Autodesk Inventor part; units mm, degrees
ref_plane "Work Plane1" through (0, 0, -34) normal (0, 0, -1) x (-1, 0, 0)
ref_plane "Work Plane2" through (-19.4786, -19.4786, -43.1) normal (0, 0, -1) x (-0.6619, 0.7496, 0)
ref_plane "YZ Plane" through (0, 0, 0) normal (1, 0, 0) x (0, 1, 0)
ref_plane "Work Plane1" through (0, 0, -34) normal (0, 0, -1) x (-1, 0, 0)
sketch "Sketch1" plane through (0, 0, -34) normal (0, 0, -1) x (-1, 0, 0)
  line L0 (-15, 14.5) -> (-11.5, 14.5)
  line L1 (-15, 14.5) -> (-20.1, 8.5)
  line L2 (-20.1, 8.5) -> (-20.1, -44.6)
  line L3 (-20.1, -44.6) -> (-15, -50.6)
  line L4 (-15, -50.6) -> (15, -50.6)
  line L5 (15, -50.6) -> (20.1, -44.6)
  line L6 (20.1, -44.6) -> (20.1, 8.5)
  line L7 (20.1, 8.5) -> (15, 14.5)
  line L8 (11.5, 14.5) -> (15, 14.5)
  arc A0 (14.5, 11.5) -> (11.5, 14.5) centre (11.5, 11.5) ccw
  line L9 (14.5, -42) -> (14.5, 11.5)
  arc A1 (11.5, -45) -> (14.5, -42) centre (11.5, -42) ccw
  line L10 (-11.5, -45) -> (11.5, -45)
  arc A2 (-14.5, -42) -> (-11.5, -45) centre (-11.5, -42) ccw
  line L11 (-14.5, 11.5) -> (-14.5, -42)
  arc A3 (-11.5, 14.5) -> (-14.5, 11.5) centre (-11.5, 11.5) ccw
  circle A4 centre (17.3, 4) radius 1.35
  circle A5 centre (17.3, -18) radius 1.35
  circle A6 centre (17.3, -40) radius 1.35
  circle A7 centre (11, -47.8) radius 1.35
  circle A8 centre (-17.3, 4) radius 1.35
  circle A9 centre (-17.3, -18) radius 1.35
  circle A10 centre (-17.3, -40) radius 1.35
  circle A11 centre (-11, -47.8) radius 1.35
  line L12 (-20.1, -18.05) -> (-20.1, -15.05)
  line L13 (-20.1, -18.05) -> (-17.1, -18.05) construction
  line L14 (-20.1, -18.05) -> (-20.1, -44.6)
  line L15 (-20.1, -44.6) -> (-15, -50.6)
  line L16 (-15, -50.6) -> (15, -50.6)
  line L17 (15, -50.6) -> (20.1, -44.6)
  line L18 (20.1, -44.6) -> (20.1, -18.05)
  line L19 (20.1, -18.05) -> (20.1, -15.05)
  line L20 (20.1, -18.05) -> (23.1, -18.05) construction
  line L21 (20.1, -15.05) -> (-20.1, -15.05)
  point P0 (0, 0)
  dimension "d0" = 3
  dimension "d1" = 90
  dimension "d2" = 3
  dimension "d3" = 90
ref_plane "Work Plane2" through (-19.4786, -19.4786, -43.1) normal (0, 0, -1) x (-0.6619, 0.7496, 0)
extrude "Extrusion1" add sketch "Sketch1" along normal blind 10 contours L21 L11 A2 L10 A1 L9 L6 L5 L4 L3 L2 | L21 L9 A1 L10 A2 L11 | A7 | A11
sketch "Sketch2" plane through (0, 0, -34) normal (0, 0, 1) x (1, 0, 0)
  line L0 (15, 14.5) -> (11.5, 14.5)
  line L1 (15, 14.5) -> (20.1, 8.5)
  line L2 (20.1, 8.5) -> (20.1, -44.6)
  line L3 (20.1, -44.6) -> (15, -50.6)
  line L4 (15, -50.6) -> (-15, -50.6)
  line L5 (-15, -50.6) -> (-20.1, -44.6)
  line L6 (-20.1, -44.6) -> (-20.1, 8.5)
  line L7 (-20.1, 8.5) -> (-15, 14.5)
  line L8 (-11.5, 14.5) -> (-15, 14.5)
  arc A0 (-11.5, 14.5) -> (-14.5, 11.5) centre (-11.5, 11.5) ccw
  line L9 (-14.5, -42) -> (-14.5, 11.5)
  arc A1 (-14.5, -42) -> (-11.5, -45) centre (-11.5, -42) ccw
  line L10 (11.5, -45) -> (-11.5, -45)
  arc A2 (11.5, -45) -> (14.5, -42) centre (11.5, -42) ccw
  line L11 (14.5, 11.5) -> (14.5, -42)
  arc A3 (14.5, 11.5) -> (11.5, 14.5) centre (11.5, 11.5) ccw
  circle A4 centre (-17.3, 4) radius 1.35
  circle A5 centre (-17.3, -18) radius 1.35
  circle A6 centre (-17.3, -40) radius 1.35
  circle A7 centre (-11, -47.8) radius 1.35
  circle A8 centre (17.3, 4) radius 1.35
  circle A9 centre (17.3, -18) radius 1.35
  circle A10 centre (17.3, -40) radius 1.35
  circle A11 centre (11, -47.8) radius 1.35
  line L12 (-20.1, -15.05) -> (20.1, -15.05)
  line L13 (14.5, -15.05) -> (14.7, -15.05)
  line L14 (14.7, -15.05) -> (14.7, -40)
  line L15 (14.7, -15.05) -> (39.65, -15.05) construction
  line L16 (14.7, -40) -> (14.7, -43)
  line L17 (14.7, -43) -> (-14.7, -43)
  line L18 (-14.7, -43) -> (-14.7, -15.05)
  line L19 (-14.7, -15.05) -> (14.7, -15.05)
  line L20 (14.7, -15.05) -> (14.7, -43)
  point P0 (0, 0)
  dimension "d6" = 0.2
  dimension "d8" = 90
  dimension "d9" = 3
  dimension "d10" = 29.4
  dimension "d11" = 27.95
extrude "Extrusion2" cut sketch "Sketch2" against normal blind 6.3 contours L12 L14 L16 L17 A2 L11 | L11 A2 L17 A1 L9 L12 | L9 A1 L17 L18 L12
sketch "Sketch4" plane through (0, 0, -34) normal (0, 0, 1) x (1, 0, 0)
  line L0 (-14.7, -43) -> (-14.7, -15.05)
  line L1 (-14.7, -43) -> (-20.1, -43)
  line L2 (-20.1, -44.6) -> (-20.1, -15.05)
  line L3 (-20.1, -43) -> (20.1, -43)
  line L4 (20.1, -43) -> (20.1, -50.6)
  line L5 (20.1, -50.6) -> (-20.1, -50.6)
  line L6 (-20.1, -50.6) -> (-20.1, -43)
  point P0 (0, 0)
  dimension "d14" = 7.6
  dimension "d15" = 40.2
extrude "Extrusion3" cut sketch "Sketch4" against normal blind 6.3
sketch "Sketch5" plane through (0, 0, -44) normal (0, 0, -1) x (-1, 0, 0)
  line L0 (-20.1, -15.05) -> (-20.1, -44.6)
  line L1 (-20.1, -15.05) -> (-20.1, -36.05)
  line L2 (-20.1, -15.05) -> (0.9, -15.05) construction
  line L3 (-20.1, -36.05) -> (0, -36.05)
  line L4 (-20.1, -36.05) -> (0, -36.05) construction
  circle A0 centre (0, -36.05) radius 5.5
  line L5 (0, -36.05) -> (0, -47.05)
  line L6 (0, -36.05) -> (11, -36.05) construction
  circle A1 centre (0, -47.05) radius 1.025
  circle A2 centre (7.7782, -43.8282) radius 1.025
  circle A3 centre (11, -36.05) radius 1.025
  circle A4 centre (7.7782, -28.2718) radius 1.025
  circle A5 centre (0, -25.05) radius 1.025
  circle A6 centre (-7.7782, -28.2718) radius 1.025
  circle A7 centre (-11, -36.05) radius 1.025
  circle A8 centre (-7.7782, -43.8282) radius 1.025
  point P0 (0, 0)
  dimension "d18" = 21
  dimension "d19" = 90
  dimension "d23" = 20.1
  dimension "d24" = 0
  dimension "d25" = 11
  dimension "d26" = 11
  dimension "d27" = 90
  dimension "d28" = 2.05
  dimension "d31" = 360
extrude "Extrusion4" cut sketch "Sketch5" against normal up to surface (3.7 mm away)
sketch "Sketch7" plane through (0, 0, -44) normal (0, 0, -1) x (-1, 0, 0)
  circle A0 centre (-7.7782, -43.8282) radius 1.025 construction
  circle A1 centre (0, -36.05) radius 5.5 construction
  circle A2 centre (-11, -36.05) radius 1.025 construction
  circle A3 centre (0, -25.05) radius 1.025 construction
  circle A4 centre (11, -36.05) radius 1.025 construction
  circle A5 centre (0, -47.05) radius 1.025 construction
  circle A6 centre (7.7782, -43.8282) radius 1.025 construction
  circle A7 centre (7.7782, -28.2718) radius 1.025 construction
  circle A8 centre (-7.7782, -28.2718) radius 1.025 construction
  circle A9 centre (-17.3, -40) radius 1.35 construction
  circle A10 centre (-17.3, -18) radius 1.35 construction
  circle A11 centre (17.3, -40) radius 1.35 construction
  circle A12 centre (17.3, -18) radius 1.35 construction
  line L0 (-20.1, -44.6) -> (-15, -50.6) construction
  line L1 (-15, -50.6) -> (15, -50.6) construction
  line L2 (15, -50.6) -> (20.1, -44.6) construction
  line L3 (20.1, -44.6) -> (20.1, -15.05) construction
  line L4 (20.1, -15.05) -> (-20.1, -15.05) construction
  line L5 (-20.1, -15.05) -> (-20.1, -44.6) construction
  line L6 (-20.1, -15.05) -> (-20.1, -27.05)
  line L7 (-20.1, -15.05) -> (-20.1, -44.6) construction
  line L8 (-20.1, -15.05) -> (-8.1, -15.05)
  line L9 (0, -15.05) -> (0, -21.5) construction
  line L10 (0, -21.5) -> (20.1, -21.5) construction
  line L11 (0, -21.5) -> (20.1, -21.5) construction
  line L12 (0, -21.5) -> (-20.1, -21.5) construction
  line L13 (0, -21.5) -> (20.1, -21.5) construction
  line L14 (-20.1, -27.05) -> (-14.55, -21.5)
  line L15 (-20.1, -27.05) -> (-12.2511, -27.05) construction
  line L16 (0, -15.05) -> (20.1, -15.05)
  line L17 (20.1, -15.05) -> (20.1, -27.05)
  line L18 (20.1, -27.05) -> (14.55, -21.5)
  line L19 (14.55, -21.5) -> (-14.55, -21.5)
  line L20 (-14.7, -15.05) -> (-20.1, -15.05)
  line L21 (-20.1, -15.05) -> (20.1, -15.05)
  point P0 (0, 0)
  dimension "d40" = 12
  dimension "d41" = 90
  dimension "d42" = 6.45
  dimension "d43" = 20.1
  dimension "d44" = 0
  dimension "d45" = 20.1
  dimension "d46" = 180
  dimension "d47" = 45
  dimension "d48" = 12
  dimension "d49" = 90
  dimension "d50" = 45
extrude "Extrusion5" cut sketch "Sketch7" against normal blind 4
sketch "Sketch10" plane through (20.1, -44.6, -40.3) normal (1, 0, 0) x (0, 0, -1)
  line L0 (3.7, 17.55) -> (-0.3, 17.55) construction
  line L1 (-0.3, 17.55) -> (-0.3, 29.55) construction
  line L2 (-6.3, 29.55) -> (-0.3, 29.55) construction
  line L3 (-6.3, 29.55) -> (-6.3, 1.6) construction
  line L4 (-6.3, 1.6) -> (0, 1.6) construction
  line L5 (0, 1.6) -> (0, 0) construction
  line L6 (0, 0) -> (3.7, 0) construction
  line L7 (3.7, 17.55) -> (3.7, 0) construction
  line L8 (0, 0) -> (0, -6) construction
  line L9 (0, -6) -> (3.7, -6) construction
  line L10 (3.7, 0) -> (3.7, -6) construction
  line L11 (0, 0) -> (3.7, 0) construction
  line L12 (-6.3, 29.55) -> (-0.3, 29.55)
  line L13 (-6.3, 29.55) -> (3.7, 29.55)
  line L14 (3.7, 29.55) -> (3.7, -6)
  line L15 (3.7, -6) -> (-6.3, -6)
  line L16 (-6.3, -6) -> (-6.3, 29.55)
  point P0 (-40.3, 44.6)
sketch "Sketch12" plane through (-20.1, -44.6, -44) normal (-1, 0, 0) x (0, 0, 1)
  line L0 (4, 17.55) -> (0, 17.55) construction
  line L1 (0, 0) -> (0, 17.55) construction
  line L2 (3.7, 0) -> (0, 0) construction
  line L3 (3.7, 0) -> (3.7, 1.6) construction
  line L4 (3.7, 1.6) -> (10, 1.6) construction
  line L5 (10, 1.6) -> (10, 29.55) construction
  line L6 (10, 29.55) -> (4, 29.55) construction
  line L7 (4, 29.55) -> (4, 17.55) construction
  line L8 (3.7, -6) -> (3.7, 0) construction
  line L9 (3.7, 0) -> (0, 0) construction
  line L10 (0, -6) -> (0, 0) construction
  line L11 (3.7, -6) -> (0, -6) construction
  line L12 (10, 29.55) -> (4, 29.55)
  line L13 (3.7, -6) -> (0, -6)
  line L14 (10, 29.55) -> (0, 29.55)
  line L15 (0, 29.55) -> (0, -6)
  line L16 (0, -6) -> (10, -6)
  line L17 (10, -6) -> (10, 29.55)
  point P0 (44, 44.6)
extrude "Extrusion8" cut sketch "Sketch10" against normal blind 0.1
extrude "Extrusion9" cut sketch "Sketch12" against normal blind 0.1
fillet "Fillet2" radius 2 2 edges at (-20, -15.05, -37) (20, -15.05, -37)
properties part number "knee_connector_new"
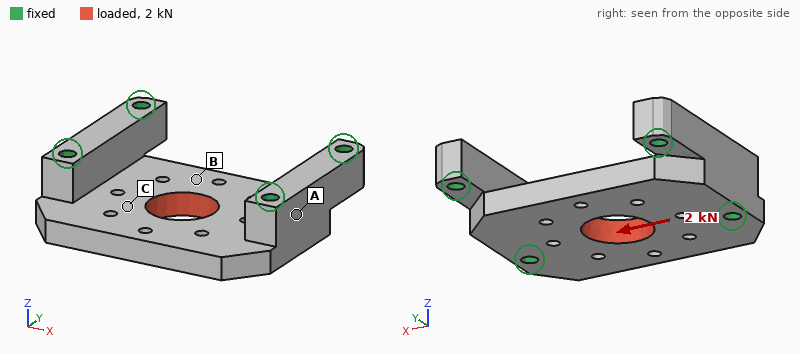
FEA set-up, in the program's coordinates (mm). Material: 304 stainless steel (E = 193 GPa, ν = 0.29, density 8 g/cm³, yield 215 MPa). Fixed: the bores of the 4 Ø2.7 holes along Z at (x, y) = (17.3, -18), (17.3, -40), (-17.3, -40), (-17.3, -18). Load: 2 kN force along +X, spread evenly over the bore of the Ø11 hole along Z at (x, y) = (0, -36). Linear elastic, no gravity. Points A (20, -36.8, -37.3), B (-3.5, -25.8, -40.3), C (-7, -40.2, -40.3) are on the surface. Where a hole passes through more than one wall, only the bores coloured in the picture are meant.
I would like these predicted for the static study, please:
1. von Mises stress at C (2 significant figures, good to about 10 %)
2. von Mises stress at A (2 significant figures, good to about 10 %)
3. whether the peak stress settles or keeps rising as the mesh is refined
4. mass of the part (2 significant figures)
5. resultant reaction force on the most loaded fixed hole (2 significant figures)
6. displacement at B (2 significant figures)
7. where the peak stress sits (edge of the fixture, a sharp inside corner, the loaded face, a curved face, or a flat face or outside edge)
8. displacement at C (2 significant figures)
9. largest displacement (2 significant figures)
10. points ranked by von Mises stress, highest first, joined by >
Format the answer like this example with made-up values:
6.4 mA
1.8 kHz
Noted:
22 MPa
9.3 MPa
keeps rising
42 g
890 N
1.9 µm
a sharp inside corner
1.2 µm
2.5 µm
C > A > B
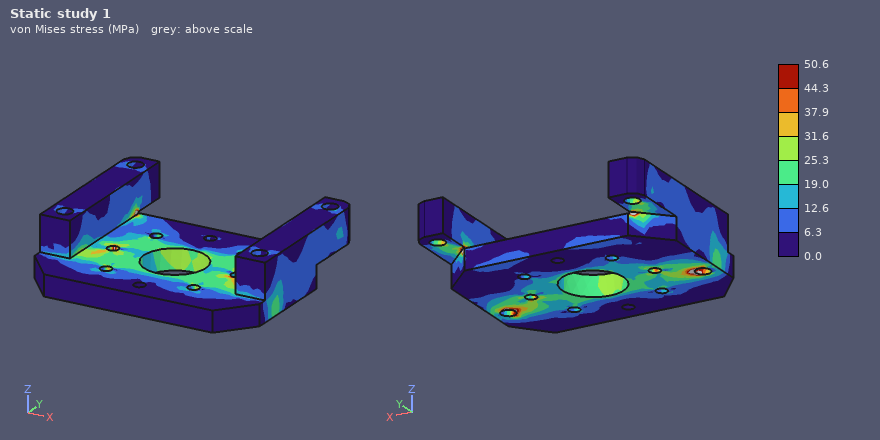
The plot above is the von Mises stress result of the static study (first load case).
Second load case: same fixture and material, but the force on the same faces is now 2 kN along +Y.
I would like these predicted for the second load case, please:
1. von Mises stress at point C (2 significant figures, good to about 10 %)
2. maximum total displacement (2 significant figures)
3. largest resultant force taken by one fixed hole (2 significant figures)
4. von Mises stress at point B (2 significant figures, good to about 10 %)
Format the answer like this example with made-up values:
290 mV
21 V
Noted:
19 MPa
3.7 µm
850 N
11 MPa
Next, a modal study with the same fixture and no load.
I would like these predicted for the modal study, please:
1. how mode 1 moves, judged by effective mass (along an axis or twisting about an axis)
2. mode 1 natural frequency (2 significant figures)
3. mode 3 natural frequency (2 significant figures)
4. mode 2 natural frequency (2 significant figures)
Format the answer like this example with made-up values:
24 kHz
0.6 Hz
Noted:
along Z
14 kHz
29 kHz
15 kHz
